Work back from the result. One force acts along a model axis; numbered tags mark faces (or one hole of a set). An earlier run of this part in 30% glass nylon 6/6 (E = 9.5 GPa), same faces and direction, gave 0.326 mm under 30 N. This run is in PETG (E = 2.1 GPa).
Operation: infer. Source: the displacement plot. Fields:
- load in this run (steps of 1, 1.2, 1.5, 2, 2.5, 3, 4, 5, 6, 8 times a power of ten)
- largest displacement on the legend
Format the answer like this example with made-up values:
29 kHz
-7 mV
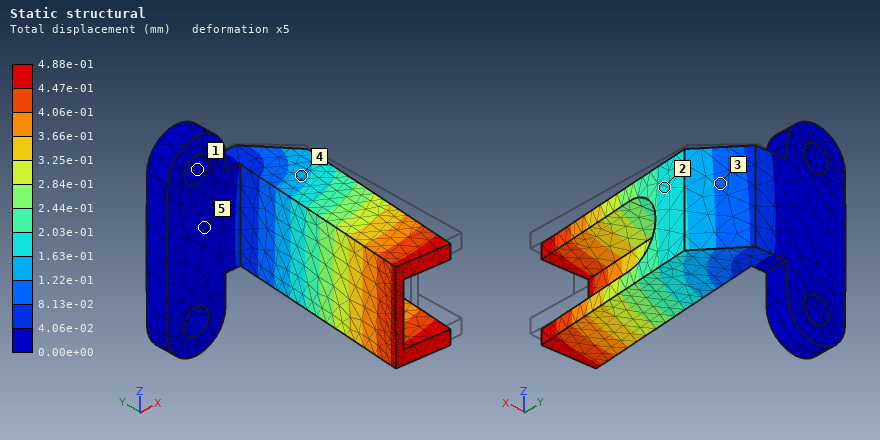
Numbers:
10 N
4.88e-01 mm
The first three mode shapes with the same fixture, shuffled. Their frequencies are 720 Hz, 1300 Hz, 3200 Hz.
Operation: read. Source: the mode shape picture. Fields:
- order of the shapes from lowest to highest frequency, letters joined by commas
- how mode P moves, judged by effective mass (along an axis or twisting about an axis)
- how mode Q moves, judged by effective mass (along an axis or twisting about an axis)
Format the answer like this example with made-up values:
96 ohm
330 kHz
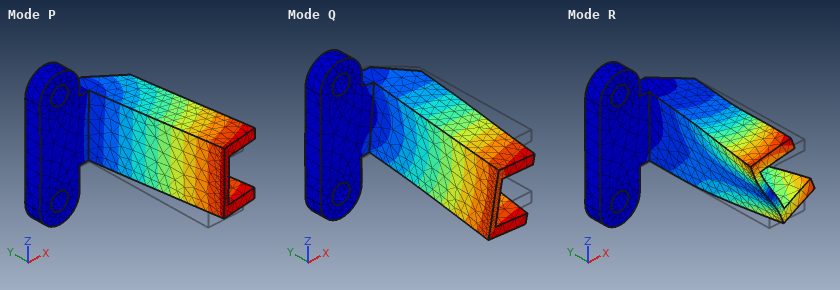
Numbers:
P, Q, R
along X
along Z
